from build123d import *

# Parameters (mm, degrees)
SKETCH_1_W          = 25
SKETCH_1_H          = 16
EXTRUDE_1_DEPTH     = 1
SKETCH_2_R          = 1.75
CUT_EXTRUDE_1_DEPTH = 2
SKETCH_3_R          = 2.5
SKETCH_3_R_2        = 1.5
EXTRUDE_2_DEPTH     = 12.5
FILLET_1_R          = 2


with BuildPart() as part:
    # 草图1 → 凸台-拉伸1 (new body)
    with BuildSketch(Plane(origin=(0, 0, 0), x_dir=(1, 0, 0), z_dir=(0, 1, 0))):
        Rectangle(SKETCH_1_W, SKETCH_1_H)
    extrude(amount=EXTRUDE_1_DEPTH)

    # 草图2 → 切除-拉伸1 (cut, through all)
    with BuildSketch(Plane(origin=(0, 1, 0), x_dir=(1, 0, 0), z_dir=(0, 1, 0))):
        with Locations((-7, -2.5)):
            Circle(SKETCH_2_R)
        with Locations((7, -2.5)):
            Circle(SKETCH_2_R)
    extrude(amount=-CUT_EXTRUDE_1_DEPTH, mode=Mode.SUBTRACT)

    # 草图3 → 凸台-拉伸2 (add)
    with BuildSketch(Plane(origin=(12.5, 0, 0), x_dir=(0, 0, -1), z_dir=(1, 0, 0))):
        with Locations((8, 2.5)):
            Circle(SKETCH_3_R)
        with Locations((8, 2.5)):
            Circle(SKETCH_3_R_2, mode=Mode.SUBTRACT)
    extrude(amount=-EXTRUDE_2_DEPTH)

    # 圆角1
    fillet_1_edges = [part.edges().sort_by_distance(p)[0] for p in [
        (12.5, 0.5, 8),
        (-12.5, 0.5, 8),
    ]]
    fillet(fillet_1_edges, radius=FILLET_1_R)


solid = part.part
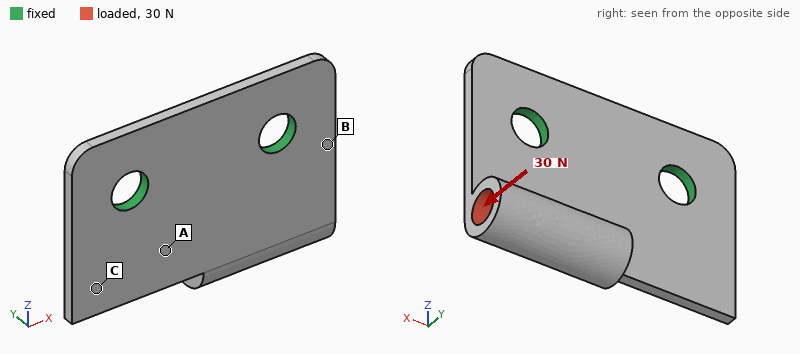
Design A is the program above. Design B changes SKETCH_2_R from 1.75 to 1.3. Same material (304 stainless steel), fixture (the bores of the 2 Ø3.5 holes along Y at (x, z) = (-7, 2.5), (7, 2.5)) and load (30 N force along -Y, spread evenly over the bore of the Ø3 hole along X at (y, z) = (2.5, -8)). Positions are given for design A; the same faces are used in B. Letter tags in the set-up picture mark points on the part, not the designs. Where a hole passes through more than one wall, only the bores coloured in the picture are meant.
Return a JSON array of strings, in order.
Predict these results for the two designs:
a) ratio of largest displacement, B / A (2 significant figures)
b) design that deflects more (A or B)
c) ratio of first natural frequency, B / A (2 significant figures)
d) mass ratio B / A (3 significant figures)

["1.2", "B", "0.93", "1.02"]
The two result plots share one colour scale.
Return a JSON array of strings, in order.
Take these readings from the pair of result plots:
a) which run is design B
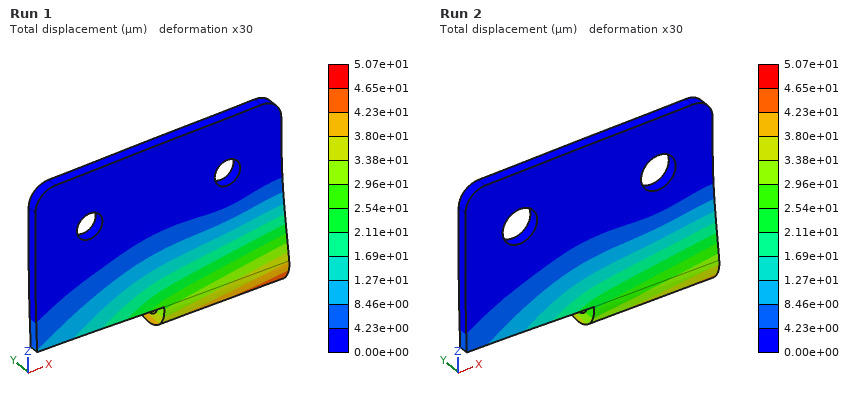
["Run 1"]
